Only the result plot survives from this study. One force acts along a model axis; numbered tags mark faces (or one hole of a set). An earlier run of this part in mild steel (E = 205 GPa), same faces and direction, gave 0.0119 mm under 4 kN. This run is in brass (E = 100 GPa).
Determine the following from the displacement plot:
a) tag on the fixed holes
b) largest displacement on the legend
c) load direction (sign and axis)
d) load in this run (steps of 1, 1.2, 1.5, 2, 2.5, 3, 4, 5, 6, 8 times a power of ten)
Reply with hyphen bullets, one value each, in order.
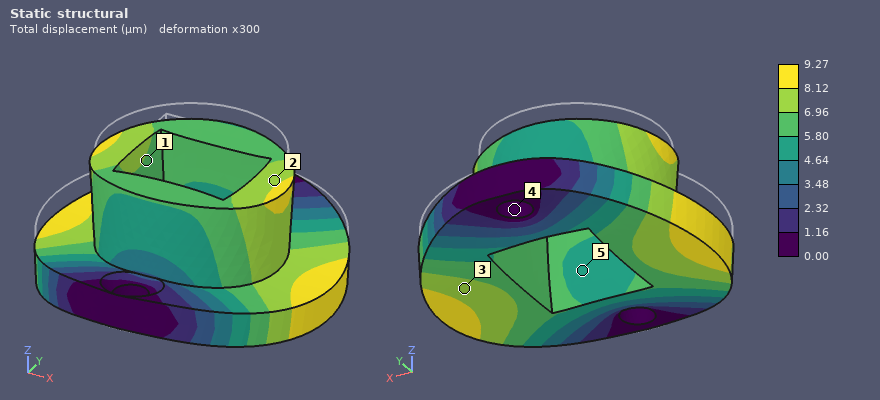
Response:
- 4
- 9.27 µm
- -Z
- 1.5 kN
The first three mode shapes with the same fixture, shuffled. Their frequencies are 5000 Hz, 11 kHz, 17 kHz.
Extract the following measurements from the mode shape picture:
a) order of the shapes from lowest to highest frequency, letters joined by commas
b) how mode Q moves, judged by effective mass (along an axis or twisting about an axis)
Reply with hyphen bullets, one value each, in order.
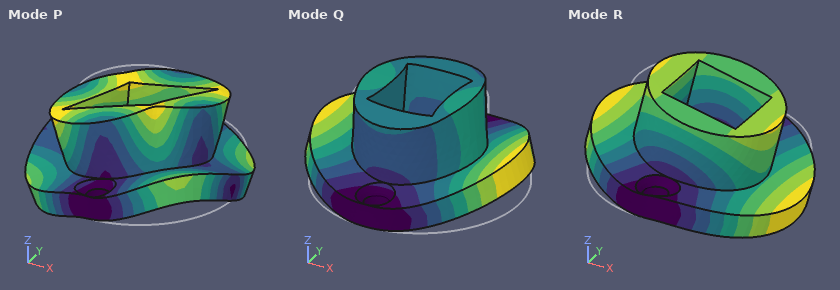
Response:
- R, Q, P
- along Z
